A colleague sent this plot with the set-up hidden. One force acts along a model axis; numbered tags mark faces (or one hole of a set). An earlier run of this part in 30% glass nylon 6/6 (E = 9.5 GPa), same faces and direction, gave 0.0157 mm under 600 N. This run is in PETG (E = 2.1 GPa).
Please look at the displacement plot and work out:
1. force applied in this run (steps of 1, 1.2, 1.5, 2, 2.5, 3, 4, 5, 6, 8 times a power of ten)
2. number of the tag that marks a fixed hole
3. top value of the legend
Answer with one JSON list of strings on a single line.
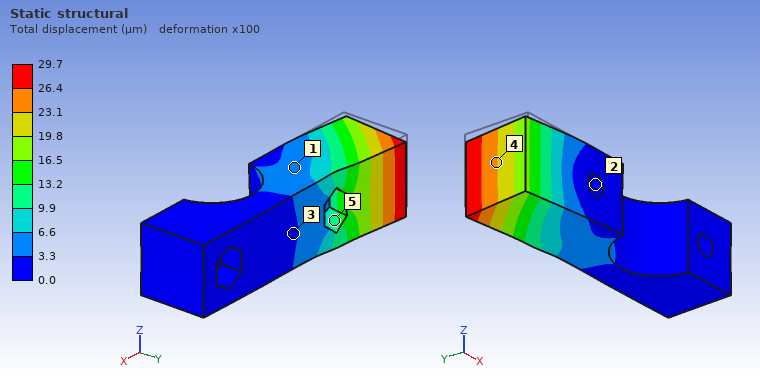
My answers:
["250 N", "2", "29.7 µm"]
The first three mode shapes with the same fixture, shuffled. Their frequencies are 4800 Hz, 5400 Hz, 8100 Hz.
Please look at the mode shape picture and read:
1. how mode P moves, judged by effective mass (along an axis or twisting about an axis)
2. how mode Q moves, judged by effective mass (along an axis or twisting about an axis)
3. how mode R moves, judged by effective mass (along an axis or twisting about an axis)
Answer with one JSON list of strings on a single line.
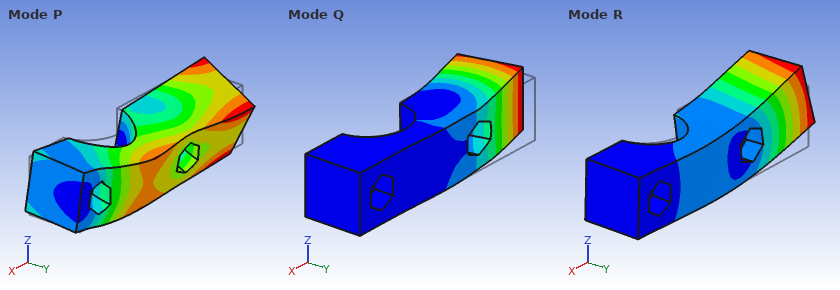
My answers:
["along Z", "along Y", "along Z"]
